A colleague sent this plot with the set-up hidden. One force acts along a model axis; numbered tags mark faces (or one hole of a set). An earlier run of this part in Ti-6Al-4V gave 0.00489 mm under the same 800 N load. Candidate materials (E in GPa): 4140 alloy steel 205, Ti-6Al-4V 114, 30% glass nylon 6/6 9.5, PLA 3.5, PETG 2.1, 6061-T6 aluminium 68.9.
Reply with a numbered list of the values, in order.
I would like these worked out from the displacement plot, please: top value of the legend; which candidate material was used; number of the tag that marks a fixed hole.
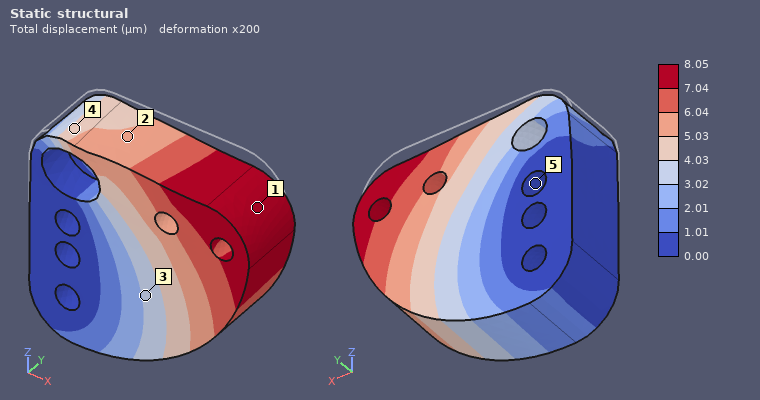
1. 8.05 µm
2. 6061-T6 aluminium
3. 5
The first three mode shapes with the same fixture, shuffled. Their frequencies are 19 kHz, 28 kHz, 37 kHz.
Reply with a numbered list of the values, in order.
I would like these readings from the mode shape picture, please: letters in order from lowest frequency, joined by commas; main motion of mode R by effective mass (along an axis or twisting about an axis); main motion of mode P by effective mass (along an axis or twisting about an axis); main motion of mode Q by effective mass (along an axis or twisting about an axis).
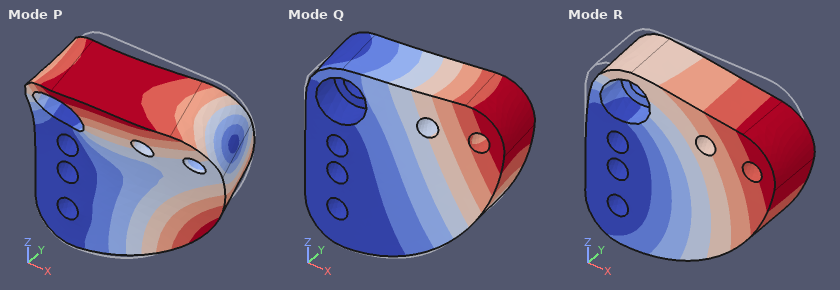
1. Q, R, P
2. along Z
3. twisting about X
4. along Y
